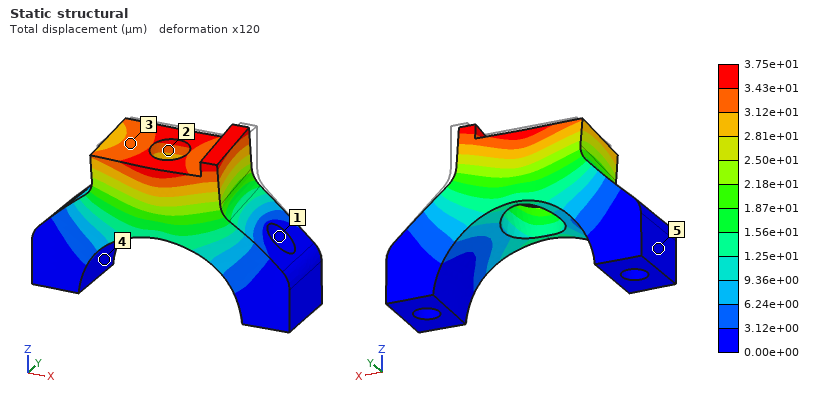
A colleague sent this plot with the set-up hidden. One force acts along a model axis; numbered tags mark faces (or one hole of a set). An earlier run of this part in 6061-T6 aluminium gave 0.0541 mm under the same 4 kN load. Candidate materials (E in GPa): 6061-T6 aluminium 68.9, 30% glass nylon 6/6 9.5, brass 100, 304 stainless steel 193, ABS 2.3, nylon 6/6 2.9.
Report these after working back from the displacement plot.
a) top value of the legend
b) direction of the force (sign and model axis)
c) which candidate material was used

3.75e+01 µm
-Y
brass
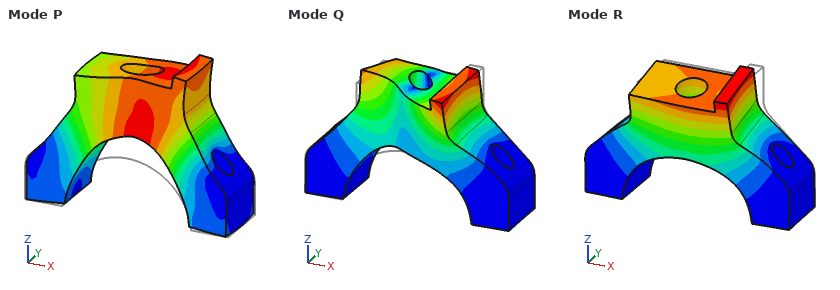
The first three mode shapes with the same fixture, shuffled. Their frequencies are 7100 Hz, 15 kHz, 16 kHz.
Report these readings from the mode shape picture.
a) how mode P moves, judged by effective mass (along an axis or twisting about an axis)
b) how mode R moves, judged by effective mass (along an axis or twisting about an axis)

along Z
along Y
